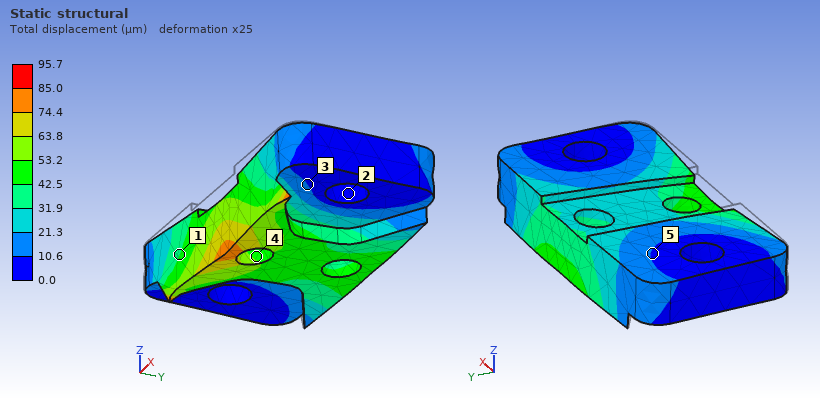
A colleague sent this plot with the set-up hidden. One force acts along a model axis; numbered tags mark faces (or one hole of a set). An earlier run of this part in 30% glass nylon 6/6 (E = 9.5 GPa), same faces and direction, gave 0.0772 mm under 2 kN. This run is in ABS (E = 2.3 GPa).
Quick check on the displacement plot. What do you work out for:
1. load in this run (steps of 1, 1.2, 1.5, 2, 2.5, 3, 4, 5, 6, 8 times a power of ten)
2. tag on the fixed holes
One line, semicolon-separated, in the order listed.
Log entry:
600 N; 2
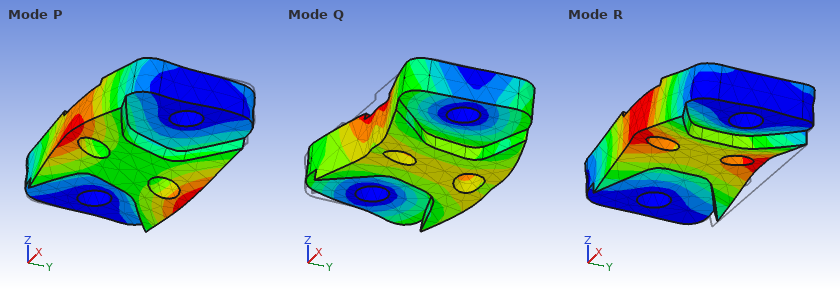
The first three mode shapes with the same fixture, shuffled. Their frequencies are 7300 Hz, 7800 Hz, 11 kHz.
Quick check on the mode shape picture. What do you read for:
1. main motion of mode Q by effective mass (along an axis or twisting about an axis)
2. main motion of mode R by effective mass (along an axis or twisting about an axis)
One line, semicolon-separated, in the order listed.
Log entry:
along Y; along Z
